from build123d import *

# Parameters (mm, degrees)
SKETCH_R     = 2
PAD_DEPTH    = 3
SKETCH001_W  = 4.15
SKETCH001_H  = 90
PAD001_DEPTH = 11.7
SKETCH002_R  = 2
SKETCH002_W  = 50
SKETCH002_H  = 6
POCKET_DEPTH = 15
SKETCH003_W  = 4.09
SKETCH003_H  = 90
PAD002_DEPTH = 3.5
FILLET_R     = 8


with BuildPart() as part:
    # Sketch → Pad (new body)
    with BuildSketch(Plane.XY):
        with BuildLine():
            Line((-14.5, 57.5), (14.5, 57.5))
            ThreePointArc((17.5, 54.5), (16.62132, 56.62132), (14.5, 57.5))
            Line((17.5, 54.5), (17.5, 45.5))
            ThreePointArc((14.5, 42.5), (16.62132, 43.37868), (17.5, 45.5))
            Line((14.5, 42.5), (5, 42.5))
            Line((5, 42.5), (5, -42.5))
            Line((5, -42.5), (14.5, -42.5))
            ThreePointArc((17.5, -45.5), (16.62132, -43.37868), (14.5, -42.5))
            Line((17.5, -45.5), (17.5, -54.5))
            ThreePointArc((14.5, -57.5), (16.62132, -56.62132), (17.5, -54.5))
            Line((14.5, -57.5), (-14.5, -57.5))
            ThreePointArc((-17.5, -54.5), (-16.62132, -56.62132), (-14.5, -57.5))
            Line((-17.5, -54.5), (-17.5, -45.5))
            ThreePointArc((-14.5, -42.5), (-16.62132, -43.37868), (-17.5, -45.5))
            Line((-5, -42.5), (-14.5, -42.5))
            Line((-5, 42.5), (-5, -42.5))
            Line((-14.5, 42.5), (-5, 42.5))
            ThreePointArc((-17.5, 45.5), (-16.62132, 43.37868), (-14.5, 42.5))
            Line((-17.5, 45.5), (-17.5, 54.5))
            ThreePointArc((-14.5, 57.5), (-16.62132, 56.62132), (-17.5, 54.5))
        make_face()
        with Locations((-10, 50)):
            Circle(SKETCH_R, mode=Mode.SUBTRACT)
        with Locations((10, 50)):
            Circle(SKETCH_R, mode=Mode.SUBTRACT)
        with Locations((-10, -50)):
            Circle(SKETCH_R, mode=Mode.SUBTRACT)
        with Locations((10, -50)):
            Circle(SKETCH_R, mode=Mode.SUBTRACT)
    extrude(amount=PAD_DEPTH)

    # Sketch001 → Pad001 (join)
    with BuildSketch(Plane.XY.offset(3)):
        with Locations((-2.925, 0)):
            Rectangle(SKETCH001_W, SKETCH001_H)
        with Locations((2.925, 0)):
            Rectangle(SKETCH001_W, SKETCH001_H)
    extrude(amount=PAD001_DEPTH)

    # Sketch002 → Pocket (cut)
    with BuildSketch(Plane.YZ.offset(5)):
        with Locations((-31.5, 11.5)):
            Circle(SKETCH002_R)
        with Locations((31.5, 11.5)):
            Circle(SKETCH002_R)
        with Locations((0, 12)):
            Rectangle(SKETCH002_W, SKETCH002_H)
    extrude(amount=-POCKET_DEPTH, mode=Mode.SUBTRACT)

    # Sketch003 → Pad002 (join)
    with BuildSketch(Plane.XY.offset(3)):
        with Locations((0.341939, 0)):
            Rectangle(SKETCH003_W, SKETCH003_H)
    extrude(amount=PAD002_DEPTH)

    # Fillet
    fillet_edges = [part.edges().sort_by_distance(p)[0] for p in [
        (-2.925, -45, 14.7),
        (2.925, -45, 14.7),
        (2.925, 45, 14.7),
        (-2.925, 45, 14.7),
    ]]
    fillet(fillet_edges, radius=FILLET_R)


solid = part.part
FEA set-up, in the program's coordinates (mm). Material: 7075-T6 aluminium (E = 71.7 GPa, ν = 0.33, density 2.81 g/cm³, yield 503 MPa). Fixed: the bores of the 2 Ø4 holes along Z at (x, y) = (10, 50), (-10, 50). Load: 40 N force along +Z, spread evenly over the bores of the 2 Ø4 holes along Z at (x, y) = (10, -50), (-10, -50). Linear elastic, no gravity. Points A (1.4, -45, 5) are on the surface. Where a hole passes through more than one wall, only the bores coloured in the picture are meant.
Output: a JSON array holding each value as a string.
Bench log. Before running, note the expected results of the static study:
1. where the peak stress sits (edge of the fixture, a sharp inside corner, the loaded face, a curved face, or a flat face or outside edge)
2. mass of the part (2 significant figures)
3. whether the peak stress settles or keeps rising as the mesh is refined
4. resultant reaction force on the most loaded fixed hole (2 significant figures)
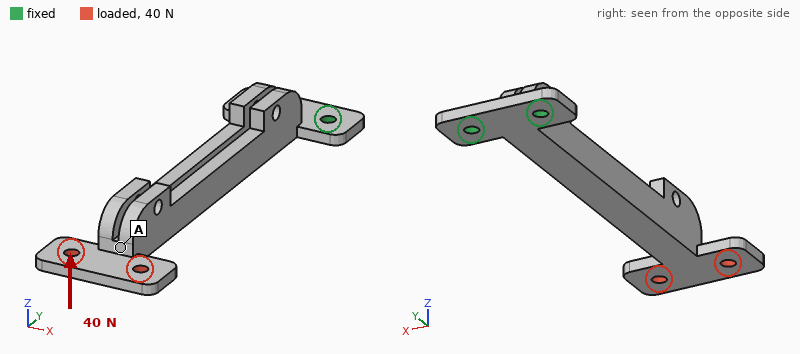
["edge of the fixture", "34 g", "keeps rising", "38 N"]
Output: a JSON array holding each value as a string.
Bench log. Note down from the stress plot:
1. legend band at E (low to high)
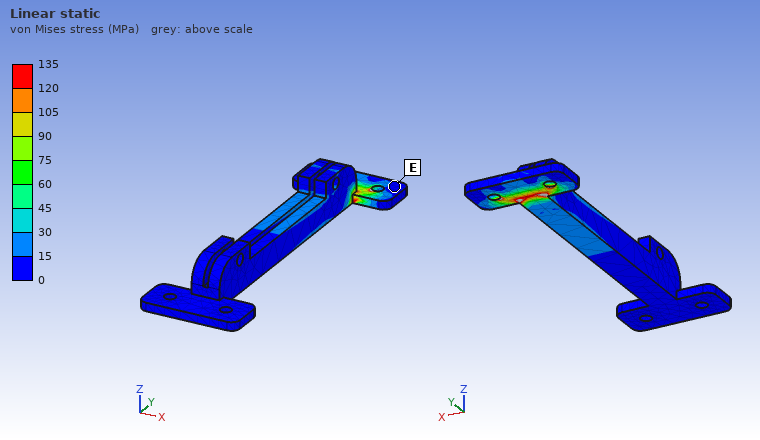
["0 to 15 MPa"]
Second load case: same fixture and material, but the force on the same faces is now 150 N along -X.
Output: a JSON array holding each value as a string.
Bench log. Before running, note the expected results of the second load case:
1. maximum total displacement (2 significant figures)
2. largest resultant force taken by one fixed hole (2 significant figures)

["1.2 mm", "800 N"]
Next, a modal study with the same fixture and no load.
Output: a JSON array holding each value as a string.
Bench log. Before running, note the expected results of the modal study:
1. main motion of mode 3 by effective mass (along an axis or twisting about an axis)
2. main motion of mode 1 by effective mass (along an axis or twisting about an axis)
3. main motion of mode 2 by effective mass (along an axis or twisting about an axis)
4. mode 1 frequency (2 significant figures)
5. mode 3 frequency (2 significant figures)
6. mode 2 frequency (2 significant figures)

["twisting about Y", "along Z", "along X", "280 Hz", "2700 Hz", "600 Hz"]
